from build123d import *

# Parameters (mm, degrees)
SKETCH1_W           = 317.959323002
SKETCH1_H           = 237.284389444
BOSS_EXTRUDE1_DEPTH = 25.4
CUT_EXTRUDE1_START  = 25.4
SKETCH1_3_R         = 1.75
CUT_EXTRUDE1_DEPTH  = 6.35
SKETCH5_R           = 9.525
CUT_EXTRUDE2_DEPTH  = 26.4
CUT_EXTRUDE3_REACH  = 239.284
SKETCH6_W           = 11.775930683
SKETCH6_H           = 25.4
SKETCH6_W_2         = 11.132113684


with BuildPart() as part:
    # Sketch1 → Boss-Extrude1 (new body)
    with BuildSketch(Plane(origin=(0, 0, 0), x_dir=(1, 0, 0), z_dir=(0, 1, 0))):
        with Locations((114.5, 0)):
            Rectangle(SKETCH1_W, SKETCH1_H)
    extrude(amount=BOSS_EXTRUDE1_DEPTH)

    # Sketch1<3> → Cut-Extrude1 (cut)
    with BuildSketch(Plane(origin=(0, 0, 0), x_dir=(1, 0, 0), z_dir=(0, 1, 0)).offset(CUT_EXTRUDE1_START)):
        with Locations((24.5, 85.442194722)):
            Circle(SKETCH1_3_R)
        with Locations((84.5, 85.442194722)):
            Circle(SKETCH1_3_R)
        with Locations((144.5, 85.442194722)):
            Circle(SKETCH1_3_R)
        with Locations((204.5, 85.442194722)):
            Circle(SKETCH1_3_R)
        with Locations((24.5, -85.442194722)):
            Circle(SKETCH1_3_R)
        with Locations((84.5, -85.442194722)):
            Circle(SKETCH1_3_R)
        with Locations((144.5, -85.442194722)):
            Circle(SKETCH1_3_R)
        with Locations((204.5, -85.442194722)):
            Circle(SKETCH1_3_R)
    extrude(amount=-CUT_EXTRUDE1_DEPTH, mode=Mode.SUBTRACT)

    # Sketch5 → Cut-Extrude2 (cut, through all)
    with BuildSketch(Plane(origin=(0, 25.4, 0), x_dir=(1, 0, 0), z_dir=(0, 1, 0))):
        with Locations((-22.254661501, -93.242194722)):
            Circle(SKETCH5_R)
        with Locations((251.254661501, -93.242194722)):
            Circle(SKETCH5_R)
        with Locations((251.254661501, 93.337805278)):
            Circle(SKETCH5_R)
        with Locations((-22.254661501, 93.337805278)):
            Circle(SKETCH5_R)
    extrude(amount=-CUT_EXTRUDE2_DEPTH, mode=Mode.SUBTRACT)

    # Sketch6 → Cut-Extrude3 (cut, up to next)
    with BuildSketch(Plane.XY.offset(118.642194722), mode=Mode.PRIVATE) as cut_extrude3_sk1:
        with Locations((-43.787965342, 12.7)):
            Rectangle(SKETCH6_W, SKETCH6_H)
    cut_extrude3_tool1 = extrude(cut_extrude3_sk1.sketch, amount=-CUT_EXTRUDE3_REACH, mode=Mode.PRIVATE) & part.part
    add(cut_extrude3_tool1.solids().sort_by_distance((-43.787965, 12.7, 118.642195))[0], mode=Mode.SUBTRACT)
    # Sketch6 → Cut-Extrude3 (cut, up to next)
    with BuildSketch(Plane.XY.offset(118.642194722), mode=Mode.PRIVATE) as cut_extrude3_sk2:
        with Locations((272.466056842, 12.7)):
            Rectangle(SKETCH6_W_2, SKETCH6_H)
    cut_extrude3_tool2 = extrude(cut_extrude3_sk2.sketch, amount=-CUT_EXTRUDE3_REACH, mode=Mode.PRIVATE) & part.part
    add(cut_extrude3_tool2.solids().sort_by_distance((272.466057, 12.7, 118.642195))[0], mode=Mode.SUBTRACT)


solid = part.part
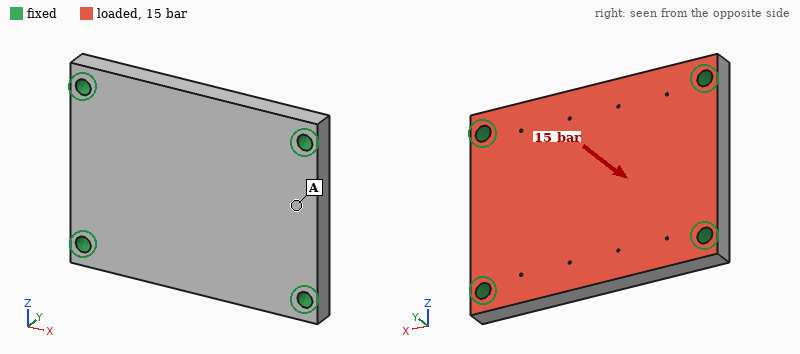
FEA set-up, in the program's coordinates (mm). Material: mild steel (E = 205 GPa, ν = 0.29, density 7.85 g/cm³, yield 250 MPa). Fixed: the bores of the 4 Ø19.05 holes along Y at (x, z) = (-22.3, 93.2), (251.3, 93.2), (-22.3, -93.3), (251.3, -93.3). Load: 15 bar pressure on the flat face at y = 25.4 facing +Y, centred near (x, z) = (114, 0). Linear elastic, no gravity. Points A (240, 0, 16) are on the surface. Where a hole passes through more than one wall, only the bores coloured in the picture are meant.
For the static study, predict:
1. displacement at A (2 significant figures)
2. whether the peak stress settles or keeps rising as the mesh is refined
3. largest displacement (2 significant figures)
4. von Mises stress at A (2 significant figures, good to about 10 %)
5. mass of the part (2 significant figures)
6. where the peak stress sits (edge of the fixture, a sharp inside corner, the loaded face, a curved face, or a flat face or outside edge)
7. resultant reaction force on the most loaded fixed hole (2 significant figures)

0.038 mm
keeps rising
0.13 mm
27 MPa
14 kg
edge of the fixture
27 kN
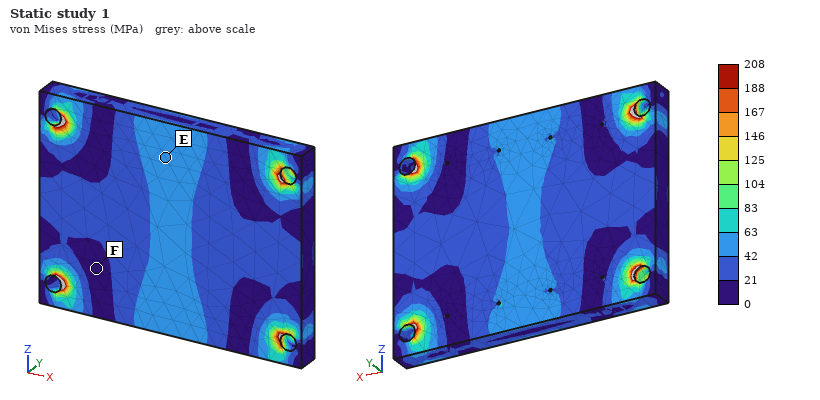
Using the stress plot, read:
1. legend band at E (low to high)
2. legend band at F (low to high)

42 to 63 MPa
0 to 21 MPa
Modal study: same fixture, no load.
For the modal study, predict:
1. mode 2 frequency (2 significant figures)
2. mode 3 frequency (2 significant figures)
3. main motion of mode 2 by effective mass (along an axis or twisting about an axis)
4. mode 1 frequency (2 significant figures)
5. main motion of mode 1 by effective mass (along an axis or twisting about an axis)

2100 Hz
3200 Hz
twisting about X
1400 Hz
along Y
